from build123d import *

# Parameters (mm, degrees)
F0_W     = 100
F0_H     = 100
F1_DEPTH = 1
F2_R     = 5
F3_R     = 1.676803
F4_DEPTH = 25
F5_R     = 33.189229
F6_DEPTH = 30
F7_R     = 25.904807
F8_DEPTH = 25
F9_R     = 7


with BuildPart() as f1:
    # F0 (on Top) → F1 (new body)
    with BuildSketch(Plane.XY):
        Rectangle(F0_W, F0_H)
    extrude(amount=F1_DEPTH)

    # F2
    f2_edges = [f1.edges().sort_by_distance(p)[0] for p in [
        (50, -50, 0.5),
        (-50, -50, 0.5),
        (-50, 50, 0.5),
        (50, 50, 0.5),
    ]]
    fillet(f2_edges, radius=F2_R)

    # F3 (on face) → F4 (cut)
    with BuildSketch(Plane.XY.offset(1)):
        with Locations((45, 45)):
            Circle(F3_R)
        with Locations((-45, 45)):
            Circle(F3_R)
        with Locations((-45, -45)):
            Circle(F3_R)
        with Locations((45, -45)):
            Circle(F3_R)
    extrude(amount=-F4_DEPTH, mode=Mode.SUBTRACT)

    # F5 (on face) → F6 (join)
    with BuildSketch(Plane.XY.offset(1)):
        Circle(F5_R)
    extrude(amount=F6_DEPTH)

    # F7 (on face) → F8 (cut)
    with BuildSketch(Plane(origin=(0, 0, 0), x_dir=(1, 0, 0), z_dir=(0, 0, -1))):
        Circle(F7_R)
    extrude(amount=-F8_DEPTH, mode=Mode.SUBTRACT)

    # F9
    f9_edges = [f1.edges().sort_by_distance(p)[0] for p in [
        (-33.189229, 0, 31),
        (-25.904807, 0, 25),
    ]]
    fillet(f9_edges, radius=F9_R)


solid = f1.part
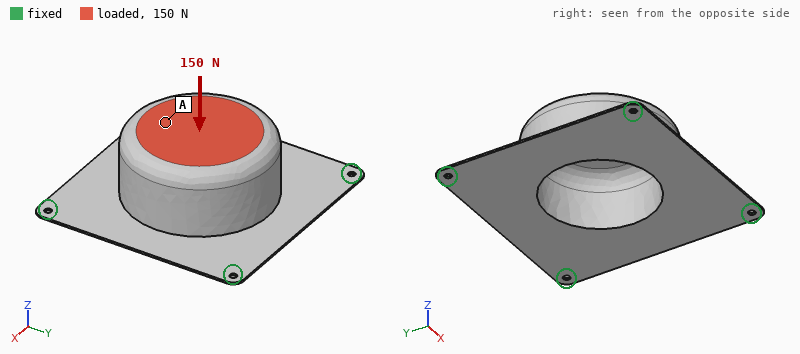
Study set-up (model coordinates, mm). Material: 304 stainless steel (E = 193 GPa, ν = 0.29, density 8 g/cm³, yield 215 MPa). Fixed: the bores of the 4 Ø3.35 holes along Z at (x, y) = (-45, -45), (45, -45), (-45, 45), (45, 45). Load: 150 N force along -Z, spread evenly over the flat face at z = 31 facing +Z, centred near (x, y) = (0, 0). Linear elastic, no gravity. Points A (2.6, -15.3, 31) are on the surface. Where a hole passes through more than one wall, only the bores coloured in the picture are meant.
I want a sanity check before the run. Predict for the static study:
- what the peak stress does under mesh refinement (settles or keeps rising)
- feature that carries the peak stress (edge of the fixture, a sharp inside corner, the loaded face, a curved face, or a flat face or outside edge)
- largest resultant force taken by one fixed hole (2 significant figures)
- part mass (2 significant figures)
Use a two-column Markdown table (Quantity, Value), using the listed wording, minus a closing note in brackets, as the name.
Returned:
| Quantity | Value |
|---|---|
| what the peak stress does under mesh refinement | keeps rising |
| feature that carries the peak stress | edge of the fixture |
| largest resultant force taken by one fixed hole | 44 N |
| part mass | 480 g |
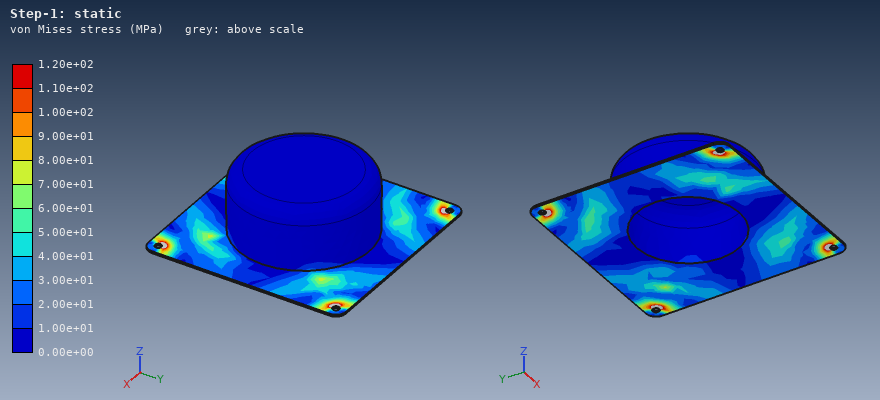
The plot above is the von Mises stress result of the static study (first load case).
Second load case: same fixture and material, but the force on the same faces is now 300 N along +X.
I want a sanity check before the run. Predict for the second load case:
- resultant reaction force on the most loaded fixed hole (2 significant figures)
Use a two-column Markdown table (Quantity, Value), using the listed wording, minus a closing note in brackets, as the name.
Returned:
| Quantity | Value |
|---|---|
| resultant reaction force on the most loaded fixed hole | 110 N |
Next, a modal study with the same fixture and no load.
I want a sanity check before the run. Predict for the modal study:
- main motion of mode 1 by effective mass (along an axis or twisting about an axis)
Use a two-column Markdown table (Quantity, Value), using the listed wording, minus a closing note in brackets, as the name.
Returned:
| Quantity | Value |
|---|---|
| main motion of mode 1 by effective mass | along Z |
